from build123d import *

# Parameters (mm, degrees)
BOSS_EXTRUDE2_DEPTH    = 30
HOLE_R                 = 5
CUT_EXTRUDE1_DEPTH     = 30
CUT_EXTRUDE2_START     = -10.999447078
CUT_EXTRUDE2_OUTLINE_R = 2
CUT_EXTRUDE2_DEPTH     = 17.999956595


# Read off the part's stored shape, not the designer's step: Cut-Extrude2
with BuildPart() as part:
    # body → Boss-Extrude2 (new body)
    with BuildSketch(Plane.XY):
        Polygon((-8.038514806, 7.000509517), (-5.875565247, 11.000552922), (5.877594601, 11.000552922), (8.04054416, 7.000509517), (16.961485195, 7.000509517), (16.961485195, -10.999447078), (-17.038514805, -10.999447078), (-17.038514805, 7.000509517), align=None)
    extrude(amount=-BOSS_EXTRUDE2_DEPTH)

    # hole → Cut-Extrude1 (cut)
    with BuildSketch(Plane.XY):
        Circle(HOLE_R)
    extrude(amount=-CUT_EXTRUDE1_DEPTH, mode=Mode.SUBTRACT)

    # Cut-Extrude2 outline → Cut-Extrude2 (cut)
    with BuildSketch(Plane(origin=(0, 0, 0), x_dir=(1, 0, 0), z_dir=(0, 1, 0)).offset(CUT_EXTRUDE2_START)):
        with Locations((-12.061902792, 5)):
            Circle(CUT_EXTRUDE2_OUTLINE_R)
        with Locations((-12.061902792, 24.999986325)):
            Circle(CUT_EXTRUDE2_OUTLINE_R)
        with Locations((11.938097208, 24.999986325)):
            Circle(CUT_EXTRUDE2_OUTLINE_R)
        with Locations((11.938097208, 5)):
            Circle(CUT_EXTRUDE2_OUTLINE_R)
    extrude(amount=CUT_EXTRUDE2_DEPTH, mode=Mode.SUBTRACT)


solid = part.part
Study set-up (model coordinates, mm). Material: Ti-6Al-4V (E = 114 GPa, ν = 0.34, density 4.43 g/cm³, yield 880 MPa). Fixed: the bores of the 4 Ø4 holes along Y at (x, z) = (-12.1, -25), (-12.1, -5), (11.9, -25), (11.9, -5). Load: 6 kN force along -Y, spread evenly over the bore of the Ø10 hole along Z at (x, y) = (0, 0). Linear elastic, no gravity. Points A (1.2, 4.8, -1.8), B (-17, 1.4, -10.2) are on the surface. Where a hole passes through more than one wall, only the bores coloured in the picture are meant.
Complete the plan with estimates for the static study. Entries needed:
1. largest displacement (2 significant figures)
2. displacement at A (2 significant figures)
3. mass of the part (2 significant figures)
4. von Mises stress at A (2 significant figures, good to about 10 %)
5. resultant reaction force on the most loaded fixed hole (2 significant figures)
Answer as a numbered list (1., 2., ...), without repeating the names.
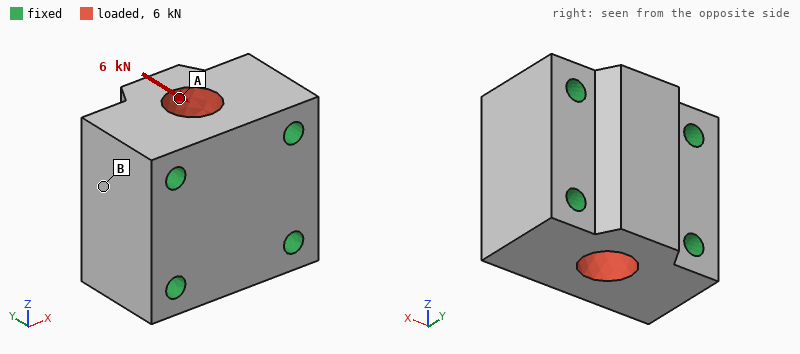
1. 1.8 µm
2. 1.6 µm
3. 74 g
4. 5.6 MPa
5. 1.5 kN
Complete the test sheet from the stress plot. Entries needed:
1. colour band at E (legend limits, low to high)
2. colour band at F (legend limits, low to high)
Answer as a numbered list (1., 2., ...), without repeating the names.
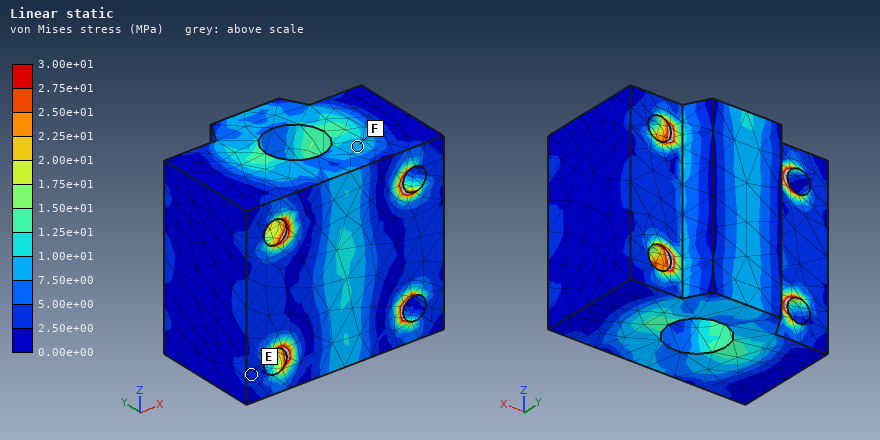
1. 2.50e+00 to 5.00e+00 MPa
2. 7.50e+00 to 1.00e+01 MPa
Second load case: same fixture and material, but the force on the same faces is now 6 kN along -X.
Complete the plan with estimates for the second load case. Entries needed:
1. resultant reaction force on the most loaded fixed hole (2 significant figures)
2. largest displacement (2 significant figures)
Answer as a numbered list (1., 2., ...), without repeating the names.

1. 1.5 kN
2. 1.0 µm
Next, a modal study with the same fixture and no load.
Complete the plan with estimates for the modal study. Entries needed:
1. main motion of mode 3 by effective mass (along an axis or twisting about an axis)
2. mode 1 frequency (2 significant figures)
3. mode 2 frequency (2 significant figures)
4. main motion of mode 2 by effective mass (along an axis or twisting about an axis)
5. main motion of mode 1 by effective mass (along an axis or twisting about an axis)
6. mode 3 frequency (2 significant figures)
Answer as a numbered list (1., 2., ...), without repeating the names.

1. along Z
2. 53 kHz
3. 56 kHz
4. along Y
5. along Z
6. 66 kHz
